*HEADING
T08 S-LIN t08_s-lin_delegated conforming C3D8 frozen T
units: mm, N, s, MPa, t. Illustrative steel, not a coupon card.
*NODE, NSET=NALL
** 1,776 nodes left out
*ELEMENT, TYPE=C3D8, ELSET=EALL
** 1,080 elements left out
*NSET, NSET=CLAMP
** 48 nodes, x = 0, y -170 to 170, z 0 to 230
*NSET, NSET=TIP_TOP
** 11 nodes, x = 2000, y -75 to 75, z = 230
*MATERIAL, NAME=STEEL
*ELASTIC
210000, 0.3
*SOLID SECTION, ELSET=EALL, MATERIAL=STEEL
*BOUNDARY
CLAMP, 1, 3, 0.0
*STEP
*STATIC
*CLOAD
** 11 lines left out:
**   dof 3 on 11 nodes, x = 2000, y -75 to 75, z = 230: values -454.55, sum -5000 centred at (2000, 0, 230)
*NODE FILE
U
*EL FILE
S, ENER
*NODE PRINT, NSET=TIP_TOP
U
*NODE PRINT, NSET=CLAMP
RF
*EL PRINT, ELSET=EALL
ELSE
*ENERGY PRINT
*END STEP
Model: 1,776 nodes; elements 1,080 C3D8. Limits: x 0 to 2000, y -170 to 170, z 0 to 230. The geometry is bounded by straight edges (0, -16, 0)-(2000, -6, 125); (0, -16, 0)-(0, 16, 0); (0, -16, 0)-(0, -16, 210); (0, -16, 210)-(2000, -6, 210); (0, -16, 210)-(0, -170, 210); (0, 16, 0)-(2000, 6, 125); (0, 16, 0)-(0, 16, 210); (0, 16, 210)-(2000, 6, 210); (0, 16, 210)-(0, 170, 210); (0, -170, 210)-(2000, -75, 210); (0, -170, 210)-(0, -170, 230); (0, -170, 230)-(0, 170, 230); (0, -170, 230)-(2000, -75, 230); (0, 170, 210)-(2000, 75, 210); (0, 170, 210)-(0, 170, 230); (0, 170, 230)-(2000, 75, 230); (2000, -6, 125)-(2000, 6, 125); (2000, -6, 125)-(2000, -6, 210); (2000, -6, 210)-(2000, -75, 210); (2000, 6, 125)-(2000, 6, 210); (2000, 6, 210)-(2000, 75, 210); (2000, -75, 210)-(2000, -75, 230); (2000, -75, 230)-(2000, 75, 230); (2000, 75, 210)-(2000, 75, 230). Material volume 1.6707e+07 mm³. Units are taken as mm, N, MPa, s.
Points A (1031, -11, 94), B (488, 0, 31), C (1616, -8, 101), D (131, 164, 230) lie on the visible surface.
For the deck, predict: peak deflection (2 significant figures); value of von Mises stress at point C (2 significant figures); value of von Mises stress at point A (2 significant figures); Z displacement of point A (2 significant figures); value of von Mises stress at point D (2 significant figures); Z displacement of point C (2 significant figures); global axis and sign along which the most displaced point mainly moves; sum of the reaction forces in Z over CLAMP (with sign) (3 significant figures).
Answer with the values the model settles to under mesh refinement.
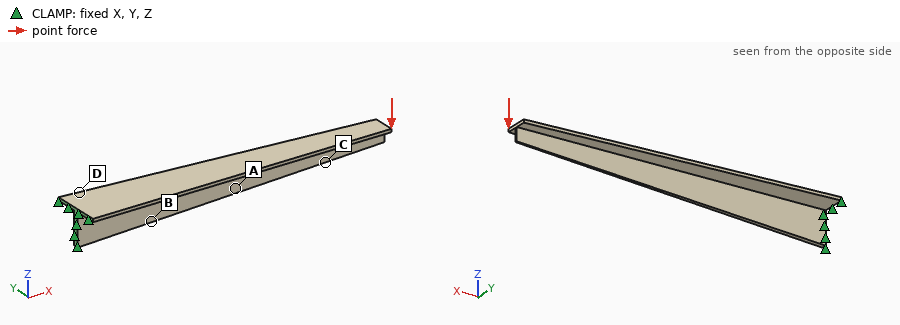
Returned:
2.1 mm
28 MPa
24 MPa
-0.46 mm
9.3 MPa
-1.3 mm
-Z
5000 N
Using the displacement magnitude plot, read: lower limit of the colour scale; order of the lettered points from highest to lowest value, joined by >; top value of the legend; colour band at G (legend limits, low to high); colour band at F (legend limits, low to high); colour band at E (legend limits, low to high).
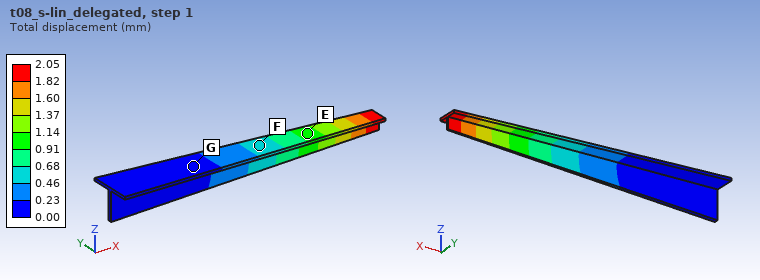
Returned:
0.00 mm
E > F > G
2.05 mm
0.00 to 0.23 mm
0.46 to 0.68 mm
0.91 to 1.14 mm
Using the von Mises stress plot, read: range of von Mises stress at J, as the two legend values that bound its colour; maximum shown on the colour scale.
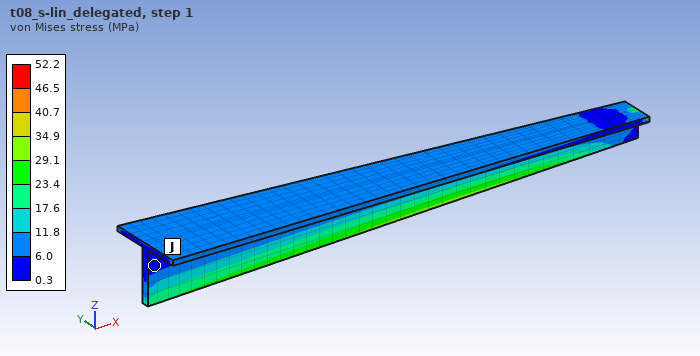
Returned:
0.3 to 6.0 MPa
52.2 MPa
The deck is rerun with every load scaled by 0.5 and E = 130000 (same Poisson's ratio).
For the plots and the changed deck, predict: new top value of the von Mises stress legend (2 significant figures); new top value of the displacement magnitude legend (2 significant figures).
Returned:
26 MPa
1.7 mm
